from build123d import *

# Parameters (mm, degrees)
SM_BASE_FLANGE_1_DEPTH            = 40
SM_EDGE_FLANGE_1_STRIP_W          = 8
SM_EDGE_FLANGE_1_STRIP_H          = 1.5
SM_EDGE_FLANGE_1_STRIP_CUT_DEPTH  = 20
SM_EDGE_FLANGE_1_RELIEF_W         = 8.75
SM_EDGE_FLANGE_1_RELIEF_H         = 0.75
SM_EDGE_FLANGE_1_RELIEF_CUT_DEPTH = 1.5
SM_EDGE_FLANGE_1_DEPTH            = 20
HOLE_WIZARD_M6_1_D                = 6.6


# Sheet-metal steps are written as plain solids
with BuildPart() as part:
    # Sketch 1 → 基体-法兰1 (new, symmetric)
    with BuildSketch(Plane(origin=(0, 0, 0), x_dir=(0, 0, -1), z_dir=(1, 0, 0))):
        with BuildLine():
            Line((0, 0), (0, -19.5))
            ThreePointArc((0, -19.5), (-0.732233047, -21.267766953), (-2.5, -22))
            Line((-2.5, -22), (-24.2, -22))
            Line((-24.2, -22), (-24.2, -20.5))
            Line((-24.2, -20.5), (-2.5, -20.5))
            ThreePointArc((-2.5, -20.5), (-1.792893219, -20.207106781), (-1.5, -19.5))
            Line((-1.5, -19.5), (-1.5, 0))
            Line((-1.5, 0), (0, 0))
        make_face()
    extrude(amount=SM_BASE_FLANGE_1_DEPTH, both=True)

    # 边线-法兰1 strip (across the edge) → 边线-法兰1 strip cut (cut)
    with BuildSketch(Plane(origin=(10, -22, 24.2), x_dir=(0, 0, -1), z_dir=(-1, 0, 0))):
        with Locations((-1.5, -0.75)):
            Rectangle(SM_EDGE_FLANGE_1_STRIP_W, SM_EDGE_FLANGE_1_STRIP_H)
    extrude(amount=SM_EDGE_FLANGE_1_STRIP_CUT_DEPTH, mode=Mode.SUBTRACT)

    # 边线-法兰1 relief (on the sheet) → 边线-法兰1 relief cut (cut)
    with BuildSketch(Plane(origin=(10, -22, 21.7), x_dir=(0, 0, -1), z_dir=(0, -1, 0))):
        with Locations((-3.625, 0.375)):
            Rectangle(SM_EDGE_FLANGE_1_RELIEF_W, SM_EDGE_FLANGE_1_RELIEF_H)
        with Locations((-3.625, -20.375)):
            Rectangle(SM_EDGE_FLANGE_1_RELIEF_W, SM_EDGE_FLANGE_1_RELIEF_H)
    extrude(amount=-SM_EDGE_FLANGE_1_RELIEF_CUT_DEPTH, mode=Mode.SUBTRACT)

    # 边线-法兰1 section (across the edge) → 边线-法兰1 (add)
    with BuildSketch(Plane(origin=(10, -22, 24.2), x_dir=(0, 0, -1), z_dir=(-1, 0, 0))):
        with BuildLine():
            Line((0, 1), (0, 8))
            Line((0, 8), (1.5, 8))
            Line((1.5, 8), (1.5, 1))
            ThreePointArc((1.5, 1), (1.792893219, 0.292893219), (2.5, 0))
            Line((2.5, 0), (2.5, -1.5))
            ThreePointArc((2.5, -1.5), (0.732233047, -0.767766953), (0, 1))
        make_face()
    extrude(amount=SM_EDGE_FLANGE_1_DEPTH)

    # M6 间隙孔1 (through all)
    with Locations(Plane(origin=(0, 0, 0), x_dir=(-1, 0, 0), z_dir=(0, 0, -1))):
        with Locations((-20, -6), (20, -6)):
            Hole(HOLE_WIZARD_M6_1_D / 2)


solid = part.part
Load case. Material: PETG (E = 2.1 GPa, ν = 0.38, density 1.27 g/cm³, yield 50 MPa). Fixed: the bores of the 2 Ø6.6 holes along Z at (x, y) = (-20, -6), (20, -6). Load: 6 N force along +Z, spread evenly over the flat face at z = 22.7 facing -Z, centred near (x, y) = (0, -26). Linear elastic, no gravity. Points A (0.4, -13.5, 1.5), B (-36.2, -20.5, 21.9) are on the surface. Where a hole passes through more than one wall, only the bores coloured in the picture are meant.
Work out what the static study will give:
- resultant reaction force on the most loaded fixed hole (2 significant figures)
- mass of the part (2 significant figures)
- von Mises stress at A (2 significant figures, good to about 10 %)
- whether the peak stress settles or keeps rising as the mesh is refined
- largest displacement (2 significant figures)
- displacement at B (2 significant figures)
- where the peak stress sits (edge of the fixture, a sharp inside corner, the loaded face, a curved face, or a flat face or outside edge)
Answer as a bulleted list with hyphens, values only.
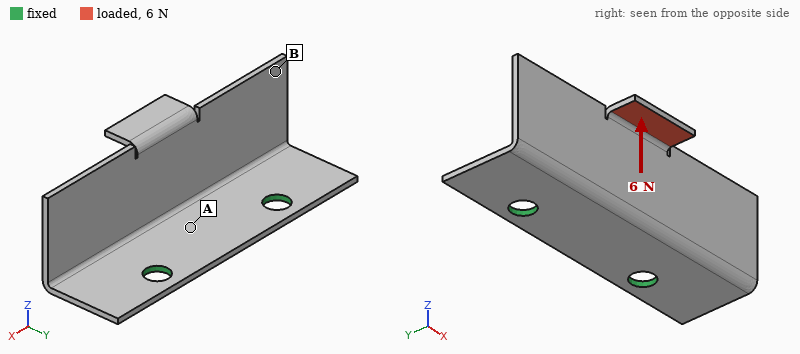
- 3.0 N
- 6.8 g
- 1.5 MPa
- keeps rising
- 1.0 mm
- 0.54 mm
- a sharp inside corner
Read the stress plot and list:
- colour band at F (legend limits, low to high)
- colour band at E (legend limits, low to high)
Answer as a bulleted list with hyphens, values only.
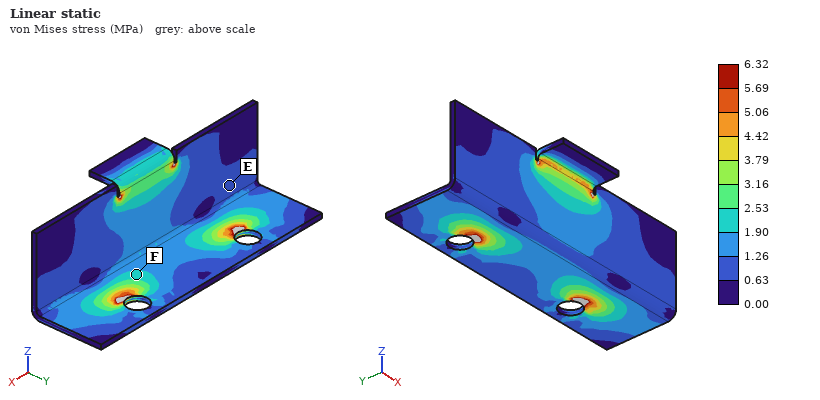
- 1.90 to 2.53 MPa
- 0.63 to 1.26 MPa
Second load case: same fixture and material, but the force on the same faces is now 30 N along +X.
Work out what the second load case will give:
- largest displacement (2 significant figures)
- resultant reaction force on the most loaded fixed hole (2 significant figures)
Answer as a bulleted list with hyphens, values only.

- 0.88 mm
- 25 N
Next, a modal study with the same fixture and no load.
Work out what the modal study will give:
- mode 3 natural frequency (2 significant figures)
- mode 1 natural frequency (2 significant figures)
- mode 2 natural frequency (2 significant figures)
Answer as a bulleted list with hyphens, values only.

- 710 Hz
- 260 Hz
- 390 Hz
